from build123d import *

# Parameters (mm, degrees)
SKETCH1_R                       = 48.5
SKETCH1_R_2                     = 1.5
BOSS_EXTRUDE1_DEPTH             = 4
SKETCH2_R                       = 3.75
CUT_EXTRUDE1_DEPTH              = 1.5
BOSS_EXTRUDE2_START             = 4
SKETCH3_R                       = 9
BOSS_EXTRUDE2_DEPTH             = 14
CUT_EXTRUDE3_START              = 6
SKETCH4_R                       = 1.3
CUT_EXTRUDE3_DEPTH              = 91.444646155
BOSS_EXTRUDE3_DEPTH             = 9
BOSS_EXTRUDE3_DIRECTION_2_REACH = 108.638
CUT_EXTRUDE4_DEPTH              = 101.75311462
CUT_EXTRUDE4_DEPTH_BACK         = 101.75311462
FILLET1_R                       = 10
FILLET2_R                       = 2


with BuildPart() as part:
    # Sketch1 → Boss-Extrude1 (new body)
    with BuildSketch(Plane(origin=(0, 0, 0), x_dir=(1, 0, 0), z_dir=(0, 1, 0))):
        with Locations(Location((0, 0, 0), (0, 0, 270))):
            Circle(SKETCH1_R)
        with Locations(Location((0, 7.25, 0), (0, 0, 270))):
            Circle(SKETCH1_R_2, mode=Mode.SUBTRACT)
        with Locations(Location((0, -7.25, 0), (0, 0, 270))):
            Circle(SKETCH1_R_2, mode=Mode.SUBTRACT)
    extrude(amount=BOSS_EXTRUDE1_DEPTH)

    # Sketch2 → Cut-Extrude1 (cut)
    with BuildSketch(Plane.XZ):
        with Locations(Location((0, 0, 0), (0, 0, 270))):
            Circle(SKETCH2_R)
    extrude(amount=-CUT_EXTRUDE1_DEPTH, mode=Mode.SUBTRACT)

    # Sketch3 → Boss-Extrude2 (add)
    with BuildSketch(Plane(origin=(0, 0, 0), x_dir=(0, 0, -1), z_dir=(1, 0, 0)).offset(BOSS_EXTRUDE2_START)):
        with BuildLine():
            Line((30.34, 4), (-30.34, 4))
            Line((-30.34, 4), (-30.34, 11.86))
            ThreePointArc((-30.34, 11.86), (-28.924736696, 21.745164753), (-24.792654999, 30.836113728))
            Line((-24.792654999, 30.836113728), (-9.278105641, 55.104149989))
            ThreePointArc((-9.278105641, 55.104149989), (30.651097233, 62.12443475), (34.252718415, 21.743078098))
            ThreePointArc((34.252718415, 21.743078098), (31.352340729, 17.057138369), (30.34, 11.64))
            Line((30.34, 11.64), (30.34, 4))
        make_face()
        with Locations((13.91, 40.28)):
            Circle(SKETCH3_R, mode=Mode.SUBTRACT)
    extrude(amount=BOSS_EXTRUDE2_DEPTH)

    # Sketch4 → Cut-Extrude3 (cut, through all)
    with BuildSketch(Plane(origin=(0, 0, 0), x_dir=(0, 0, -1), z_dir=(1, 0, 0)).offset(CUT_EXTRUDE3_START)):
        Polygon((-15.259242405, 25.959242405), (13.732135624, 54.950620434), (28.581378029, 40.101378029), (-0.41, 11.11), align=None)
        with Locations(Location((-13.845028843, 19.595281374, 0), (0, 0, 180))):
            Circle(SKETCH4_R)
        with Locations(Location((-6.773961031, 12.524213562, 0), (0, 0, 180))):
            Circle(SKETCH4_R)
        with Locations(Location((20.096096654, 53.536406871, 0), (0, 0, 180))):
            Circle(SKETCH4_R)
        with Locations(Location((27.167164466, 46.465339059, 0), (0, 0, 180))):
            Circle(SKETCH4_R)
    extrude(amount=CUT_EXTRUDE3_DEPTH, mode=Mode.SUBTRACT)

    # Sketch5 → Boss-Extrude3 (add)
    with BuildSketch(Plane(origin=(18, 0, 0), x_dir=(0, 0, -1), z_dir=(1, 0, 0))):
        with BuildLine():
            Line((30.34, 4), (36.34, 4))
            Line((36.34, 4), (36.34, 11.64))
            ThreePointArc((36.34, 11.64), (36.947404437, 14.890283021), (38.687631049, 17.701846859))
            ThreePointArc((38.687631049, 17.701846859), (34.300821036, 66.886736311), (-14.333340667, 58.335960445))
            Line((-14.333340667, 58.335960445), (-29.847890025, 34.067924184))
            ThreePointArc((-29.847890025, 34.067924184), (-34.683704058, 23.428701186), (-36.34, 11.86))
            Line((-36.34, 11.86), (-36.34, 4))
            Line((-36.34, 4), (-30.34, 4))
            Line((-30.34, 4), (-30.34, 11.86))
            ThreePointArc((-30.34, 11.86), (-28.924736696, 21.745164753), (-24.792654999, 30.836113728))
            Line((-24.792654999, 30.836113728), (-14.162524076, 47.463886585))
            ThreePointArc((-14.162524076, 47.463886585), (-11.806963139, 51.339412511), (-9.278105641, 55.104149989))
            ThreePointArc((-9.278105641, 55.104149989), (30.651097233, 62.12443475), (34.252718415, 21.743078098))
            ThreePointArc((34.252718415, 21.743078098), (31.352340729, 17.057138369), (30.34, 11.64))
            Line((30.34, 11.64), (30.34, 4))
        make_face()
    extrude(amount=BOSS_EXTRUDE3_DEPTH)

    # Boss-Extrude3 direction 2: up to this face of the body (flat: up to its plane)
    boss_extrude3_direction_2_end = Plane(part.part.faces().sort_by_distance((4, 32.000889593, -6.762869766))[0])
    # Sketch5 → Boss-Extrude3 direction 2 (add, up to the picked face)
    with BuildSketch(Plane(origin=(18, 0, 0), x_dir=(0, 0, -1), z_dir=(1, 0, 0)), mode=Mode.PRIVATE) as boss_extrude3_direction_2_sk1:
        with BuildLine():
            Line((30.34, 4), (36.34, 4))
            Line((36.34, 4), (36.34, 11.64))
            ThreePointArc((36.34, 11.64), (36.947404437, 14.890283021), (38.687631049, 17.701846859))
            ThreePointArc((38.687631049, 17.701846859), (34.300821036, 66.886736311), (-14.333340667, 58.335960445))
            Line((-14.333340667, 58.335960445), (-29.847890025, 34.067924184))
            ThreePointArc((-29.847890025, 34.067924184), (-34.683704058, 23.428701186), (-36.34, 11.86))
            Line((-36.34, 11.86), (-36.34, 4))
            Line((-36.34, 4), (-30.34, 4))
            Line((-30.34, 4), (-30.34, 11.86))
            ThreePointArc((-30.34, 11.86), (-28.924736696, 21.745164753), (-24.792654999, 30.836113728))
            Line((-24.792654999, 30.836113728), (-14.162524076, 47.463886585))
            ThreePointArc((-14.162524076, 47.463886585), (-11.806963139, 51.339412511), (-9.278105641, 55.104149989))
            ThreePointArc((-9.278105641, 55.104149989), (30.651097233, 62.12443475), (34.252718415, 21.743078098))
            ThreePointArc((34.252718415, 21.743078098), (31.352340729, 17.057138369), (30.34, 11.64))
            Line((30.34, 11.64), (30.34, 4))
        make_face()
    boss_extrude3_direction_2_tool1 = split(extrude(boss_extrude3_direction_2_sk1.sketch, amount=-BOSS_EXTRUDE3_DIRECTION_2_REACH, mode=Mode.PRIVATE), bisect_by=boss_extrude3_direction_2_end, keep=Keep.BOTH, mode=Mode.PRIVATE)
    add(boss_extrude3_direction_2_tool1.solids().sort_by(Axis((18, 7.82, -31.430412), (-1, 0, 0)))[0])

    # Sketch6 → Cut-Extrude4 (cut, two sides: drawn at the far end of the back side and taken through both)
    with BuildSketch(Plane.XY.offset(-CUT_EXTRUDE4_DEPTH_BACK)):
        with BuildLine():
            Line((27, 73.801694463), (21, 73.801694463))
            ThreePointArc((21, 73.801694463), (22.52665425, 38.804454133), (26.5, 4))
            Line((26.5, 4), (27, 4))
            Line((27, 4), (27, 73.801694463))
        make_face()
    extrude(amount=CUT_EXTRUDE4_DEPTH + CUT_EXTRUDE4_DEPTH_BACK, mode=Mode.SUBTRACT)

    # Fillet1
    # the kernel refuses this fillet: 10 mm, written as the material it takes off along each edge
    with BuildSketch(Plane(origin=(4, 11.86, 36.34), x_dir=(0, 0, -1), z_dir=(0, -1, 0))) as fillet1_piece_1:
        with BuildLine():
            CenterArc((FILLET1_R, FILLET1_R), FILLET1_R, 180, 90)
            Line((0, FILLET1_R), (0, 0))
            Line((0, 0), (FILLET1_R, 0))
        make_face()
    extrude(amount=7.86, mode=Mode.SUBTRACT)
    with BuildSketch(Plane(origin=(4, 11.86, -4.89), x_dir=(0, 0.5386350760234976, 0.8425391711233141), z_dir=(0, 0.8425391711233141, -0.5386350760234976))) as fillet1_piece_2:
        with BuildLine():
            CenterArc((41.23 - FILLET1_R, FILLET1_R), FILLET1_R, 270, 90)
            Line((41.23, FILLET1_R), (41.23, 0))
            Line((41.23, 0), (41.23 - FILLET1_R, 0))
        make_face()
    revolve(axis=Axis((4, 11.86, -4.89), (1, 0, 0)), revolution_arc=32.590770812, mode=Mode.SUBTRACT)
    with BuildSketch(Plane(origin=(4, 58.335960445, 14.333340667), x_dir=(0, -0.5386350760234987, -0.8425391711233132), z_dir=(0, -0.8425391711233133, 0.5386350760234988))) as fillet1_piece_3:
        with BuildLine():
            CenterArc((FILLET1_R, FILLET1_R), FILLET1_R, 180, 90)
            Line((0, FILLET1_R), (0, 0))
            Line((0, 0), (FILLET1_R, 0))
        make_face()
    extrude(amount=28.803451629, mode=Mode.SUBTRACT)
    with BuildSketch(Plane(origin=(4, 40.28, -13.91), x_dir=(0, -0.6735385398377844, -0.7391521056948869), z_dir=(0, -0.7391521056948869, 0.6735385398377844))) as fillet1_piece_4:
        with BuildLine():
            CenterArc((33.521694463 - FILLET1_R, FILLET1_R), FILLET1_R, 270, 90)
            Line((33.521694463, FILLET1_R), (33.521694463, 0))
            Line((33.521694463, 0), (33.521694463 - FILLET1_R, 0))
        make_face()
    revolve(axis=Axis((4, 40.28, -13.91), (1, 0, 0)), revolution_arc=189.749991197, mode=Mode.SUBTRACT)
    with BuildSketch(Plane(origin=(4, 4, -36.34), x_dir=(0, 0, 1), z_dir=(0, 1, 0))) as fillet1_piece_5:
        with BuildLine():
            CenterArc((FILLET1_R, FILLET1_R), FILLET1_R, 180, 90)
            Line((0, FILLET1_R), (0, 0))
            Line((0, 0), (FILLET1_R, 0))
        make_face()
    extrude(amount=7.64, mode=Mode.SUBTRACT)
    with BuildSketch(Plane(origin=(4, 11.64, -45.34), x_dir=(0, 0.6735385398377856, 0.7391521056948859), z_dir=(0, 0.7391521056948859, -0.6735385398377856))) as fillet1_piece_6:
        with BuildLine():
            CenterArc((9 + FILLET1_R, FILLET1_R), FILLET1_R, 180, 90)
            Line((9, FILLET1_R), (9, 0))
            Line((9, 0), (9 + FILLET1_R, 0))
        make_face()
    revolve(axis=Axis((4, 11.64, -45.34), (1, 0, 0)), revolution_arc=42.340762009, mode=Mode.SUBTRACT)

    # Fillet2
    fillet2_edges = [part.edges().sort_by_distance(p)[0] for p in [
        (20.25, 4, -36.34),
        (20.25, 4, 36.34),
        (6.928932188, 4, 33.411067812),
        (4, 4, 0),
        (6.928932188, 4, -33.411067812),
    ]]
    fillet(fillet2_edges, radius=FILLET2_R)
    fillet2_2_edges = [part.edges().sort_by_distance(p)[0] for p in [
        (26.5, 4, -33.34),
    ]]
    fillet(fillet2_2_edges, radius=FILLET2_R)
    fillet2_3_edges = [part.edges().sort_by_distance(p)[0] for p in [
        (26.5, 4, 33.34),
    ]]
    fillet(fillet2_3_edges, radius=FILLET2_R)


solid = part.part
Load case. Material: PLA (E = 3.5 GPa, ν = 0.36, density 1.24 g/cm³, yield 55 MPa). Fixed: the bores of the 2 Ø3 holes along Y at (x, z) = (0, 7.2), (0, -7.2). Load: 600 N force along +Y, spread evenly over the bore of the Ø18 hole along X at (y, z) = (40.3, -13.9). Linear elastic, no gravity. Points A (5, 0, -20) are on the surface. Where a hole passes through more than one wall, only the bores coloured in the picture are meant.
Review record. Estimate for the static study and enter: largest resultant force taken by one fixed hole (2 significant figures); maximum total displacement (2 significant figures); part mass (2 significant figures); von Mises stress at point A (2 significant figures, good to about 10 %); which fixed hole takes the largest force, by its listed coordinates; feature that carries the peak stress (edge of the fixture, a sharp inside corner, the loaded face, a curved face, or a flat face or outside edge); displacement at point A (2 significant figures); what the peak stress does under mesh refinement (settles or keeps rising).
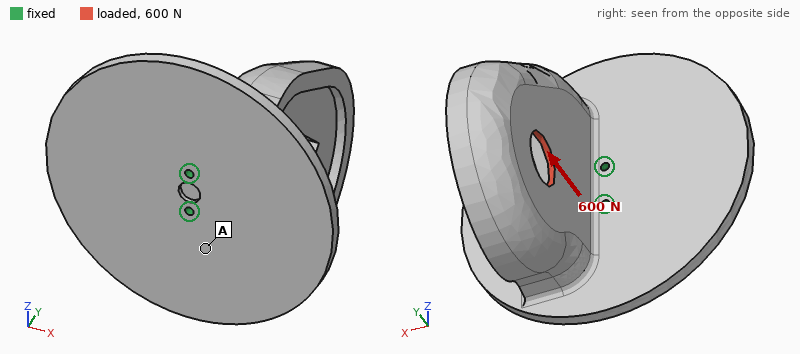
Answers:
750 N
1.2 mm
100 g
4.1 MPa
(0, -7.2)
edge of the fixture
0.28 mm
keeps rising
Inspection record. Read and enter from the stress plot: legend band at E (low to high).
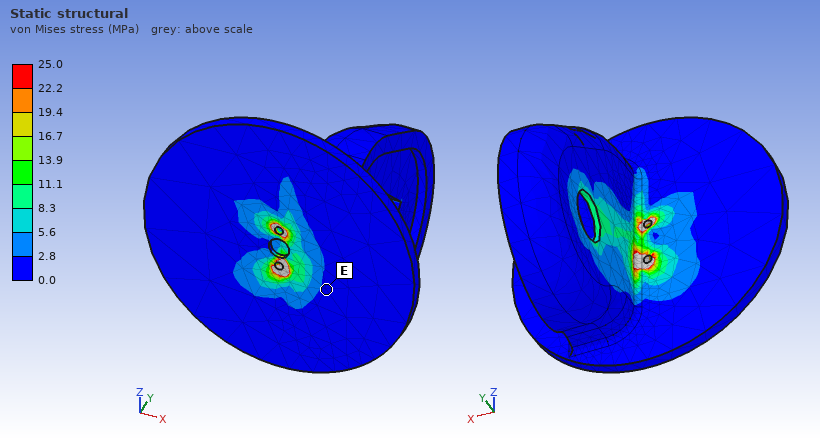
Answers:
0.0 to 2.8 MPa
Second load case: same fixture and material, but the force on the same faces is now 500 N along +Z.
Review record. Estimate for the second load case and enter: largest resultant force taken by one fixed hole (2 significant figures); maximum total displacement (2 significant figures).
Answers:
1.1 kN
1.7 mm
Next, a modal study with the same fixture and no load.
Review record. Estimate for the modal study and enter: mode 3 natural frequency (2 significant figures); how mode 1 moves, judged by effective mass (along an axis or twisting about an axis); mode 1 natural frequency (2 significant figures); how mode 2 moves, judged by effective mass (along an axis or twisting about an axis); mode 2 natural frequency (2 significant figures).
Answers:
550 Hz
along X
170 Hz
along Z
370 Hz
